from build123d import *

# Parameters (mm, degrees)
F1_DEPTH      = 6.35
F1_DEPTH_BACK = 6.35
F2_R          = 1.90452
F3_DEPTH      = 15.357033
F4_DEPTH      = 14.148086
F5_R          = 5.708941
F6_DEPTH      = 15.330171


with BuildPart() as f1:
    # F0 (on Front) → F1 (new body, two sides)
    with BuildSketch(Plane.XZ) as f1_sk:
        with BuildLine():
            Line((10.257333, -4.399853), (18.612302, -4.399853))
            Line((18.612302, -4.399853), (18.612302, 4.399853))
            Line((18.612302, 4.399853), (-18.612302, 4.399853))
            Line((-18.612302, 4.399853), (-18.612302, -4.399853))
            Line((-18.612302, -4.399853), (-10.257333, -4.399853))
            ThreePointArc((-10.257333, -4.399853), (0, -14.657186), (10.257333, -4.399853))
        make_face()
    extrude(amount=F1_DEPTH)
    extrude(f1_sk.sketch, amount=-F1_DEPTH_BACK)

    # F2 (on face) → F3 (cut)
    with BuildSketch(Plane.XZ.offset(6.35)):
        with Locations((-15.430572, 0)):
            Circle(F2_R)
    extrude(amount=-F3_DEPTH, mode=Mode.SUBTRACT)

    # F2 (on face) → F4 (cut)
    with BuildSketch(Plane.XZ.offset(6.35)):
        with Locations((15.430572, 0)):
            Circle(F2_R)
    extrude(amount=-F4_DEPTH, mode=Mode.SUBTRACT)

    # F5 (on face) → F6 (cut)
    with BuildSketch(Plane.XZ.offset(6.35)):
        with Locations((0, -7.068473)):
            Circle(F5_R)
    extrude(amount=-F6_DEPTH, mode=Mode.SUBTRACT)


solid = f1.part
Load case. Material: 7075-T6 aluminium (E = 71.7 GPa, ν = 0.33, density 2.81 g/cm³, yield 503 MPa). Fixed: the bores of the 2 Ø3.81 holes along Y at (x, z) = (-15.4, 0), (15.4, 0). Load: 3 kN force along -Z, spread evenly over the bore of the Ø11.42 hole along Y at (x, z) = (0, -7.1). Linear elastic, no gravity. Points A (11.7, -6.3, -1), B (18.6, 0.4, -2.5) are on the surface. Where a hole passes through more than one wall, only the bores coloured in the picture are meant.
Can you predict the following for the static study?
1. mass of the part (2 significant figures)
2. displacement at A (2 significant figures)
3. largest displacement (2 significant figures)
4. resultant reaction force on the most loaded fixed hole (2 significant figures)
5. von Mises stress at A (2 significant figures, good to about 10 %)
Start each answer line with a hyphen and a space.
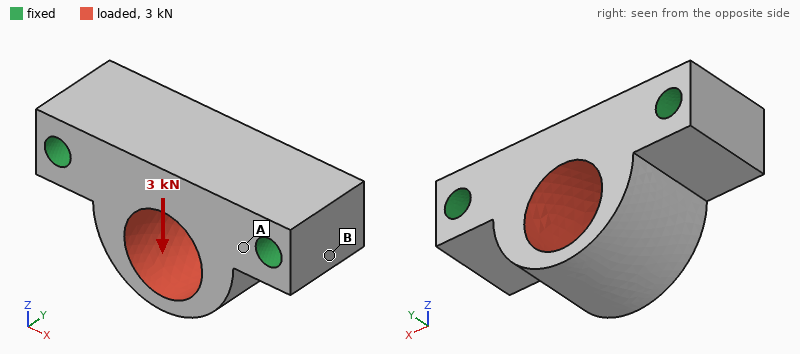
- 13 g
- 2.6 µm
- 11 µm
- 1.5 kN
- 38 MPa
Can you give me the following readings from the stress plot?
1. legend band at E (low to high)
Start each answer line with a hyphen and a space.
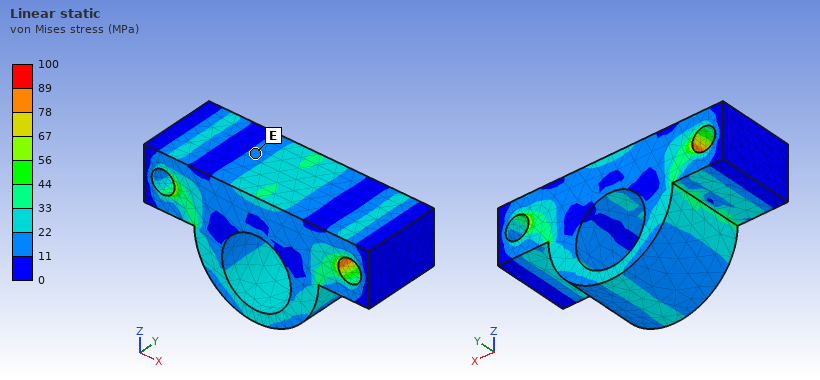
- 11 to 22 MPa
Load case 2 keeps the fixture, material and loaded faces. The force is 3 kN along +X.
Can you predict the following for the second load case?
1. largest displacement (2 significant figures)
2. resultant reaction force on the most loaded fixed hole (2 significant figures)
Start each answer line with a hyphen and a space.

- 21 µm
- 1.7 kN
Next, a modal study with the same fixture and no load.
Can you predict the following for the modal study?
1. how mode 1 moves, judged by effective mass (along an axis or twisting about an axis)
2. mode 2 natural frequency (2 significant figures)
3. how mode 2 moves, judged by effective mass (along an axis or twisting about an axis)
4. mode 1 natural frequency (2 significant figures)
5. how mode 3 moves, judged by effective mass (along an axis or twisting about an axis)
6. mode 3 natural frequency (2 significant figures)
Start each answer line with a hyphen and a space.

- along Y
- 31 kHz
- along Z
- 25 kHz
- along X
- 34 kHz
